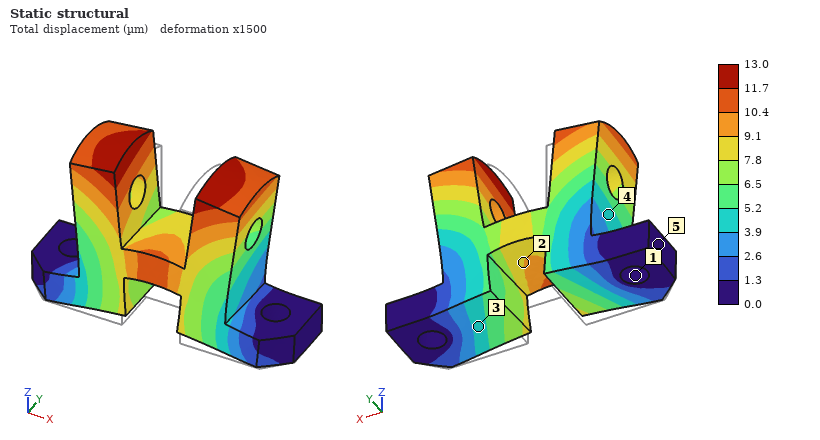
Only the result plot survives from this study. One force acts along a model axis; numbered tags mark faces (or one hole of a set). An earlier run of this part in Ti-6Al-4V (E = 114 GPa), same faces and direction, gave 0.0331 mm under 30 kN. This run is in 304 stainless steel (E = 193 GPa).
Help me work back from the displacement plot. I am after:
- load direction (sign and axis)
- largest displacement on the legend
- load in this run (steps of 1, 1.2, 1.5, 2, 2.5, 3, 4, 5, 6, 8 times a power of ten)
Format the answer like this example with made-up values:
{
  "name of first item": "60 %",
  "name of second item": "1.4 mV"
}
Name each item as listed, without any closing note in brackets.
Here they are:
{
  "load direction": "+Z",
  "largest displacement on the legend": "13.0 µm",
  "load in this run": "20 kN"
}
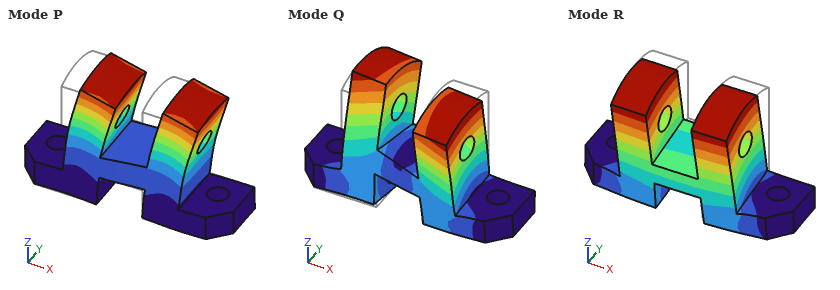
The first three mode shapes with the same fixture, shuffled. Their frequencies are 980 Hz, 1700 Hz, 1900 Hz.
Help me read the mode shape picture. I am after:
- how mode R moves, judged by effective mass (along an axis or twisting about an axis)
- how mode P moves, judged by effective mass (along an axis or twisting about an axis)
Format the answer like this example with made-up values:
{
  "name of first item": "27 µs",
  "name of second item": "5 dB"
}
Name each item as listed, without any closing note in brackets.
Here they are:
{
  "how mode R moves, judged by effective mass": "along Y",
  "how mode P moves, judged by effective mass": "along X"
}
